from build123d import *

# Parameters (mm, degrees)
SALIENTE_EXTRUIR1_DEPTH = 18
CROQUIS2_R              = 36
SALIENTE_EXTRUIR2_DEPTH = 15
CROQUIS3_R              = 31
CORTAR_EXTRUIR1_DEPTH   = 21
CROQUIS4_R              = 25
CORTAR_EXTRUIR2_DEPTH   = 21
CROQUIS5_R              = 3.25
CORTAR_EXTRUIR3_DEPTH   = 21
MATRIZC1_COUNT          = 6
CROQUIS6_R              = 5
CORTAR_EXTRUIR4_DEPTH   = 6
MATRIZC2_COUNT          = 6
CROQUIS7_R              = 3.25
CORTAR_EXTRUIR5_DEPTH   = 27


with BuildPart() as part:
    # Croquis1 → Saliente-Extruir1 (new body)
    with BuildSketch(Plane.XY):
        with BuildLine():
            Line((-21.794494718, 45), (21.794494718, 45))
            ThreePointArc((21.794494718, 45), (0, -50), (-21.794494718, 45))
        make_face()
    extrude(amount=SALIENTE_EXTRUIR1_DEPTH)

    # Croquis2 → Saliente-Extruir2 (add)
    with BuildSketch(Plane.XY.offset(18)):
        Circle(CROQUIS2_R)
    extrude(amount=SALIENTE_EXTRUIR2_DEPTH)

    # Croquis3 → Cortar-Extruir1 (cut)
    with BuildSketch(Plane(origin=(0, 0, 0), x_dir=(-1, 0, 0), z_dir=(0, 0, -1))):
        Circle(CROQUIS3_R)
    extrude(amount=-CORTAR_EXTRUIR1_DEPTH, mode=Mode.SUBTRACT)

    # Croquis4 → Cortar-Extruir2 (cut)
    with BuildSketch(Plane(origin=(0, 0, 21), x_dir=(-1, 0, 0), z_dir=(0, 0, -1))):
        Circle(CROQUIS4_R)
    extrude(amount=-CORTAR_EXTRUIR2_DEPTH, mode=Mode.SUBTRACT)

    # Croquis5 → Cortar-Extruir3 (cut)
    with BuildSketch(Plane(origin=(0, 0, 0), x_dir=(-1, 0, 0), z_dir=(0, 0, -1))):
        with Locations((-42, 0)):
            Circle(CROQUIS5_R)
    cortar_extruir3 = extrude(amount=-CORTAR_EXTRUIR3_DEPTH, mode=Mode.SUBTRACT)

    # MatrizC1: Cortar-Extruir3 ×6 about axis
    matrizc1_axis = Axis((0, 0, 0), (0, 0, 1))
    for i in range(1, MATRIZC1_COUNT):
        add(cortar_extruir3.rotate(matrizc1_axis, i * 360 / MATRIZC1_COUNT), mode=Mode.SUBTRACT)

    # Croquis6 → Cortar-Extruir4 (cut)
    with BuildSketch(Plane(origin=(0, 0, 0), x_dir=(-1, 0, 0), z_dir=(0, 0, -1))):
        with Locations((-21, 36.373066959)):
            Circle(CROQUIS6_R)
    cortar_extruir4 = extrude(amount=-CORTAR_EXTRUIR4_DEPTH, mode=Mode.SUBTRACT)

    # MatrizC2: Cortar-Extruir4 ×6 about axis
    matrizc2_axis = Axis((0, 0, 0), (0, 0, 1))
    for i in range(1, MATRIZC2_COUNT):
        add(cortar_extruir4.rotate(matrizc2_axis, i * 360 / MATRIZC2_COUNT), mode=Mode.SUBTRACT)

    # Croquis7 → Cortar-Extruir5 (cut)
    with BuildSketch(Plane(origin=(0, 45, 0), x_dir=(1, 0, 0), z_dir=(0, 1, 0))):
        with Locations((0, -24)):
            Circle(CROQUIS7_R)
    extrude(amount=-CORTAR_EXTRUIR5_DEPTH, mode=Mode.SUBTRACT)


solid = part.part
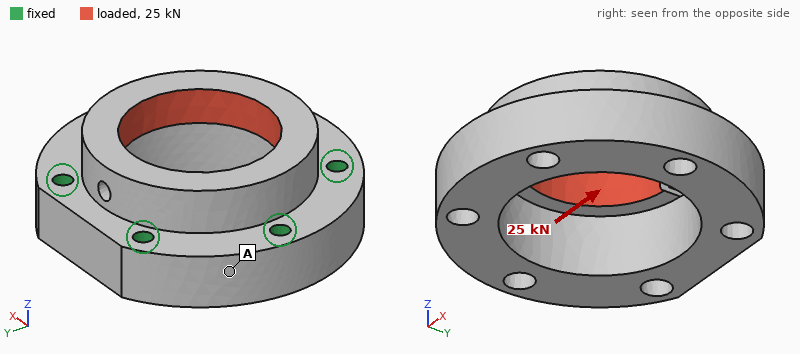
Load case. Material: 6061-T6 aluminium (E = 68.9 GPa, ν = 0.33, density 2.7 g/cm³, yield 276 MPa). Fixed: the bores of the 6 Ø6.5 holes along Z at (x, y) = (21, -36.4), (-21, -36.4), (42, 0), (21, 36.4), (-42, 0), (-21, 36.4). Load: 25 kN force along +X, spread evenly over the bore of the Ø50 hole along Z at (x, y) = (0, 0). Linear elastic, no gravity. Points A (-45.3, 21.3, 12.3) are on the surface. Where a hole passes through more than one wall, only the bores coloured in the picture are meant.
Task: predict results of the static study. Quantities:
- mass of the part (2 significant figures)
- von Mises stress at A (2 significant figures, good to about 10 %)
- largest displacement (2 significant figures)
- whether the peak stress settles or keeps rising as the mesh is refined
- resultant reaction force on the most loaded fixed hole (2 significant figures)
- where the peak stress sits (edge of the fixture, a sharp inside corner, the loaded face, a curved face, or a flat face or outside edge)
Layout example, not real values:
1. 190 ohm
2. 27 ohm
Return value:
1. 290 g
2. 7.1 MPa
3. 42 µm
4. keeps rising
5. 4.9 kN
6. a sharp inside corner
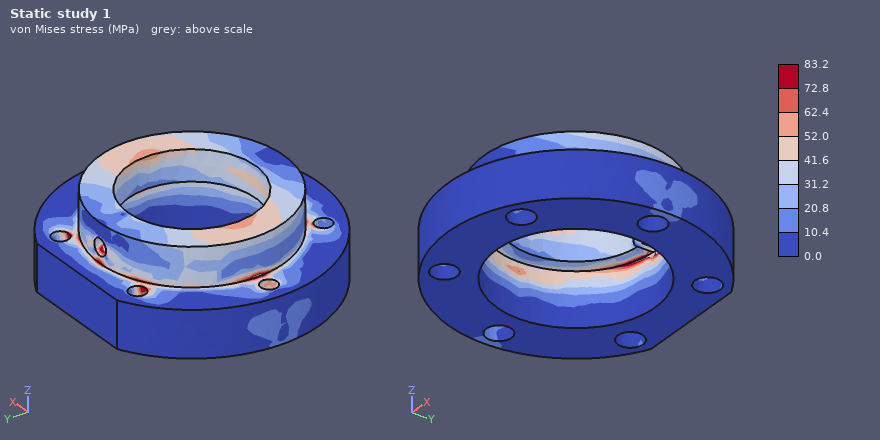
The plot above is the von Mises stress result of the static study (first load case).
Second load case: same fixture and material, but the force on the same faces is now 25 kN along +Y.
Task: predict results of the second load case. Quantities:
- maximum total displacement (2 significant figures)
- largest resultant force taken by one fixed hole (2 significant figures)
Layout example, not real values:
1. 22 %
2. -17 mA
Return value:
1. 42 µm
2. 4.7 kN
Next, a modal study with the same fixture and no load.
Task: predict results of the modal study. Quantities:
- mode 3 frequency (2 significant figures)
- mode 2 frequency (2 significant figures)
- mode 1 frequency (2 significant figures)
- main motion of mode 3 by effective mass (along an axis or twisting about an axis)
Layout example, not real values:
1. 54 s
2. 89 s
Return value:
1. 19 kHz
2. 18 kHz
3. 18 kHz
4. along X
